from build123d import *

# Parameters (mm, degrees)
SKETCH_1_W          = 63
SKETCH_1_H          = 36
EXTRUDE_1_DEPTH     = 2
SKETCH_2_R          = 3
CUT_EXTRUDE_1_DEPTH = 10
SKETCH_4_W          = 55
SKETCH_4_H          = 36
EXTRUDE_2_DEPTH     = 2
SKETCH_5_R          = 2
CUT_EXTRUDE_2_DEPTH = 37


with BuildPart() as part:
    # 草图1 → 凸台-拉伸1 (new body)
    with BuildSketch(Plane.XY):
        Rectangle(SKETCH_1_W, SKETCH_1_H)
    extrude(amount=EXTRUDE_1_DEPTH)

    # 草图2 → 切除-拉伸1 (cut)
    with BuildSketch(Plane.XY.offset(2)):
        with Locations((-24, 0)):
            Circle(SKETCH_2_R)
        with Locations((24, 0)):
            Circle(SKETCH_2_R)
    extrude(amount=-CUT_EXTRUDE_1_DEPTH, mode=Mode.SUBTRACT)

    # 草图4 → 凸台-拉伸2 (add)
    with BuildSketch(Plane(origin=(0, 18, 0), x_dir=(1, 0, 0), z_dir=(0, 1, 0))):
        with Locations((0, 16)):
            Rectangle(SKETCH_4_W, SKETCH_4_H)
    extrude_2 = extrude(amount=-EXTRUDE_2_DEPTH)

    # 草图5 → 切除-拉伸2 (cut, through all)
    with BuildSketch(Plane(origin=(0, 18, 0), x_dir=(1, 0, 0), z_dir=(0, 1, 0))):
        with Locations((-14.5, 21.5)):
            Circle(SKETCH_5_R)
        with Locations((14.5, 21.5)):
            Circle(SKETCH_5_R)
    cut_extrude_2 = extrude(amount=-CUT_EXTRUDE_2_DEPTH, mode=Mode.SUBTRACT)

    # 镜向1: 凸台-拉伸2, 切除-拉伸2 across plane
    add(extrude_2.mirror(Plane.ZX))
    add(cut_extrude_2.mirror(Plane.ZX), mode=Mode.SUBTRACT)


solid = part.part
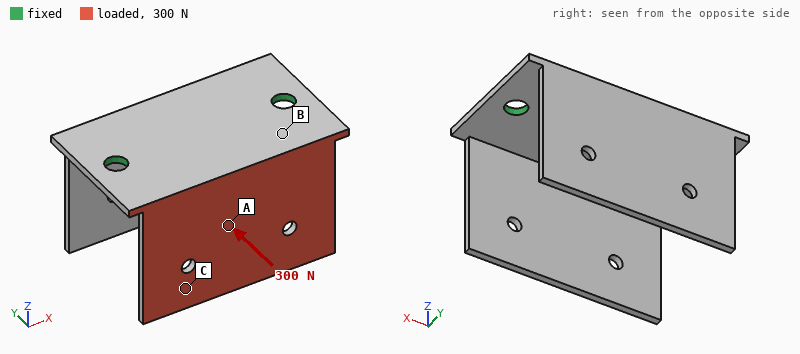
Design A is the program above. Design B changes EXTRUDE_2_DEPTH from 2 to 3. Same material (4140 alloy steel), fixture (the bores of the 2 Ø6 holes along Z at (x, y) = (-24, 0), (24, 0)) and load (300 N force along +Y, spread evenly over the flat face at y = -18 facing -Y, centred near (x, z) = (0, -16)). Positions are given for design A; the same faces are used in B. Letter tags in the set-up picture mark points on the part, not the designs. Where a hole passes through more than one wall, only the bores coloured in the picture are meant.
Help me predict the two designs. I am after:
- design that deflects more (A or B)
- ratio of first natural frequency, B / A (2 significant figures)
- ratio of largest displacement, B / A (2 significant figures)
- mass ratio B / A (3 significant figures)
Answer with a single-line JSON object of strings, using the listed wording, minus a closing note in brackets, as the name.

{"design that deflects more": "A", "ratio of first natural frequency, B / A": "0.93", "ratio of largest displacement, B / A": "0.72", "mass ratio B / A": "1.31"}
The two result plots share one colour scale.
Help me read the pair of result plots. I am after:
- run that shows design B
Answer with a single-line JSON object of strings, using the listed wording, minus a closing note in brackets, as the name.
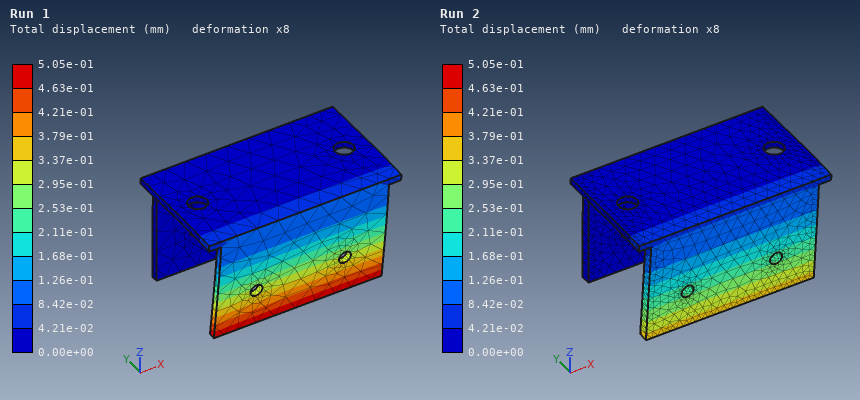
{"run that shows design B": "Run 2"}
